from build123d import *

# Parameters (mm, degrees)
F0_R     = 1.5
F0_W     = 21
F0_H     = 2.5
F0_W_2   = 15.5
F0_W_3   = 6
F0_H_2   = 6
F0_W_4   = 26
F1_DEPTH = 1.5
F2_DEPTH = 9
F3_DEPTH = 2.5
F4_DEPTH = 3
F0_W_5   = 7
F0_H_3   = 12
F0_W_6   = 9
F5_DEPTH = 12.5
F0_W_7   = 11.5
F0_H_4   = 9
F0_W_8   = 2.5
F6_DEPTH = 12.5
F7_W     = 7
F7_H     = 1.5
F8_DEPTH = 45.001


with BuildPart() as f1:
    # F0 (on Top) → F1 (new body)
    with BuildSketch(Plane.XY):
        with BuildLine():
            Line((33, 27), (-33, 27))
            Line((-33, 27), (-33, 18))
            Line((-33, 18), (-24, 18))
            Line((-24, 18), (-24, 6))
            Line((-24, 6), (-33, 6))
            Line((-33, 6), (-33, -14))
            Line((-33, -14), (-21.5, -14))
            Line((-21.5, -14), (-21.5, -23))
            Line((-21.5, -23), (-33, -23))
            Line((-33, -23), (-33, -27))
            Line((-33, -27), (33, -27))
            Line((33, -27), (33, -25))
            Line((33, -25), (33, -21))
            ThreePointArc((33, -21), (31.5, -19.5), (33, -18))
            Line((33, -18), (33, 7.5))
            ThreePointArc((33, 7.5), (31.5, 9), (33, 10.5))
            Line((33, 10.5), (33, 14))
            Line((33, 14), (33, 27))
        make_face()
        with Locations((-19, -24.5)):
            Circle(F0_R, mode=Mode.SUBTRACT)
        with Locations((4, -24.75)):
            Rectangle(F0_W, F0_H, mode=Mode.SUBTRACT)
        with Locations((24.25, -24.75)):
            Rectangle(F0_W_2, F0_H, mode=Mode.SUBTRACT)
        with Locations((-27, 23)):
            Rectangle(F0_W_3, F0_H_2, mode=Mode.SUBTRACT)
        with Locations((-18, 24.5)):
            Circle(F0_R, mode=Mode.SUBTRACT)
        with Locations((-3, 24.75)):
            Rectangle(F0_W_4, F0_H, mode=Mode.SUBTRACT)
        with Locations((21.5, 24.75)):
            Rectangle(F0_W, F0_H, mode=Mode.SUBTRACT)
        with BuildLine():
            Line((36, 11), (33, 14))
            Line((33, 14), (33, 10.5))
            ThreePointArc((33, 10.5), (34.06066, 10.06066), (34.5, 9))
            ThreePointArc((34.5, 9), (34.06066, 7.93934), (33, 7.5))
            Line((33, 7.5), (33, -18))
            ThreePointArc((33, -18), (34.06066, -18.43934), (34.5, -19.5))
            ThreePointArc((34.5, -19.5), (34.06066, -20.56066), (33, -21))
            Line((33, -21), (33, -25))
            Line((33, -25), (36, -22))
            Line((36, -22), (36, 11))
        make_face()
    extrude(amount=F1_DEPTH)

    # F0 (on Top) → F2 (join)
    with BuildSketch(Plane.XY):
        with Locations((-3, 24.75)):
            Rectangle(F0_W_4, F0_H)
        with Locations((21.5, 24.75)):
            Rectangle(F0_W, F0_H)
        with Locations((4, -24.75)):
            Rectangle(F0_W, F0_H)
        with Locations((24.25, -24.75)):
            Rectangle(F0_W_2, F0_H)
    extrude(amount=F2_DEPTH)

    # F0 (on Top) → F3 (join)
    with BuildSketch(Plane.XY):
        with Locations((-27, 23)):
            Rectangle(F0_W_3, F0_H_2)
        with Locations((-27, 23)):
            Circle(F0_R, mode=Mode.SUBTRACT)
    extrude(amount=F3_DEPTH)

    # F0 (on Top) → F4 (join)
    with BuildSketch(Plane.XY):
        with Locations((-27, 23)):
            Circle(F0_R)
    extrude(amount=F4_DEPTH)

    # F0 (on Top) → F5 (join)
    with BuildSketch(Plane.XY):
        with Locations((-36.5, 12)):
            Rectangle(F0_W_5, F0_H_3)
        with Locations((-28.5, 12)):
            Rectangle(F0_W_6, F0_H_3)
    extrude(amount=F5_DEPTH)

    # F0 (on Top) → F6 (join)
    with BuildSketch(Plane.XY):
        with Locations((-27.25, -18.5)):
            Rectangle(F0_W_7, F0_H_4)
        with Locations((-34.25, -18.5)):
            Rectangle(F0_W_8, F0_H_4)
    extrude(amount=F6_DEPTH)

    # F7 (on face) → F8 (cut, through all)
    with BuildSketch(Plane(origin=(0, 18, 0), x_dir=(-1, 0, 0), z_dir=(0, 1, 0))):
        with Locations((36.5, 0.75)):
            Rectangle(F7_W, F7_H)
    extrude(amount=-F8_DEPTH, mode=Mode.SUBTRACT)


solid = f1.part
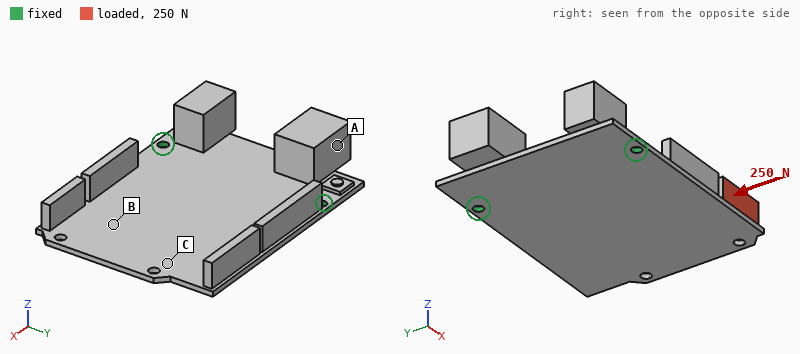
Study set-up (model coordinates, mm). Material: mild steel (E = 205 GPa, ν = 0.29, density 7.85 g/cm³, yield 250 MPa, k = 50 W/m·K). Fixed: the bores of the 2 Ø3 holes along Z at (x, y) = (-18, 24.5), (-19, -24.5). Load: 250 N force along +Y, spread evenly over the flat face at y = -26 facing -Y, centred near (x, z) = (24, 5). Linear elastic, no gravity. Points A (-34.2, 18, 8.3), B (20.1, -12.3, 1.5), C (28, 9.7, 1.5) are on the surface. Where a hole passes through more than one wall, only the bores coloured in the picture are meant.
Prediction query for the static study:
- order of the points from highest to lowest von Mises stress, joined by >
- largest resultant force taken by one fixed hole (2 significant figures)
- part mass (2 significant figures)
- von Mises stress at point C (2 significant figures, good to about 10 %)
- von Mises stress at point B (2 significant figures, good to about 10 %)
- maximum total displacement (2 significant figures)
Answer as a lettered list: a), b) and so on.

a) B > C > A
b) 260 N
c) 83 g
d) 24 MPa
e) 53 MPa
f) 0.19 mm
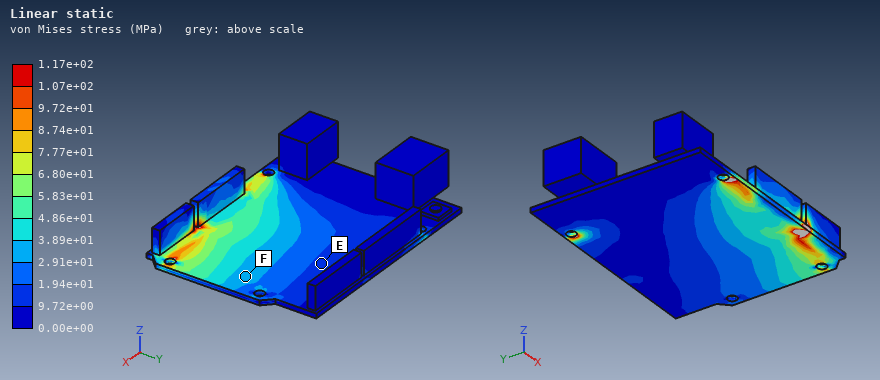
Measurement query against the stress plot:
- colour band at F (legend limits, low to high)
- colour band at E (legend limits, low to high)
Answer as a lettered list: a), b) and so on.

a) 2.91e+01 to 3.89e+01 MPa
b) 9.72e+00 to 1.94e+01 MPa
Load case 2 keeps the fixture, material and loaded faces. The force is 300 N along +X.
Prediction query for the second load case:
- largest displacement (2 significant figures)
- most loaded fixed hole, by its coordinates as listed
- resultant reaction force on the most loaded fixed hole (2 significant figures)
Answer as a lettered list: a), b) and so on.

a) 0.52 mm
b) (-19, -24.5)
c) 310 N
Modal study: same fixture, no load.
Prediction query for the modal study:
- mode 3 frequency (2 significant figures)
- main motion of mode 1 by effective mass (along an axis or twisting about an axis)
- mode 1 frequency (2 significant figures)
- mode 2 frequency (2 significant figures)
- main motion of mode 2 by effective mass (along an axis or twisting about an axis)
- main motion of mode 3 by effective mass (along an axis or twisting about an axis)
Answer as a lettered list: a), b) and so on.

a) 1100 Hz
b) along Z
c) 420 Hz
d) 960 Hz
e) twisting about X
f) along Z
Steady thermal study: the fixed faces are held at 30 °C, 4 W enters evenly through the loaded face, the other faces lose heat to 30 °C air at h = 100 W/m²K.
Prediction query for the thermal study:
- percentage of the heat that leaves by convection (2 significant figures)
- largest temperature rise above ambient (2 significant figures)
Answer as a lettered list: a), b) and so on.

a) 93 %
b) 33 K
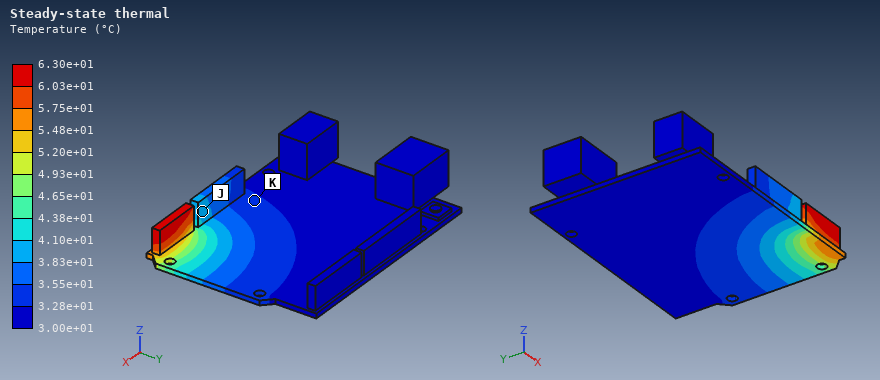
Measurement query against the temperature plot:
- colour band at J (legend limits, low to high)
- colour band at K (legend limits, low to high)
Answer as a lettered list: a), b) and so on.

a) 3.83e+01 to 4.10e+01 °C
b) 3.28e+01 to 3.55e+01 °C
